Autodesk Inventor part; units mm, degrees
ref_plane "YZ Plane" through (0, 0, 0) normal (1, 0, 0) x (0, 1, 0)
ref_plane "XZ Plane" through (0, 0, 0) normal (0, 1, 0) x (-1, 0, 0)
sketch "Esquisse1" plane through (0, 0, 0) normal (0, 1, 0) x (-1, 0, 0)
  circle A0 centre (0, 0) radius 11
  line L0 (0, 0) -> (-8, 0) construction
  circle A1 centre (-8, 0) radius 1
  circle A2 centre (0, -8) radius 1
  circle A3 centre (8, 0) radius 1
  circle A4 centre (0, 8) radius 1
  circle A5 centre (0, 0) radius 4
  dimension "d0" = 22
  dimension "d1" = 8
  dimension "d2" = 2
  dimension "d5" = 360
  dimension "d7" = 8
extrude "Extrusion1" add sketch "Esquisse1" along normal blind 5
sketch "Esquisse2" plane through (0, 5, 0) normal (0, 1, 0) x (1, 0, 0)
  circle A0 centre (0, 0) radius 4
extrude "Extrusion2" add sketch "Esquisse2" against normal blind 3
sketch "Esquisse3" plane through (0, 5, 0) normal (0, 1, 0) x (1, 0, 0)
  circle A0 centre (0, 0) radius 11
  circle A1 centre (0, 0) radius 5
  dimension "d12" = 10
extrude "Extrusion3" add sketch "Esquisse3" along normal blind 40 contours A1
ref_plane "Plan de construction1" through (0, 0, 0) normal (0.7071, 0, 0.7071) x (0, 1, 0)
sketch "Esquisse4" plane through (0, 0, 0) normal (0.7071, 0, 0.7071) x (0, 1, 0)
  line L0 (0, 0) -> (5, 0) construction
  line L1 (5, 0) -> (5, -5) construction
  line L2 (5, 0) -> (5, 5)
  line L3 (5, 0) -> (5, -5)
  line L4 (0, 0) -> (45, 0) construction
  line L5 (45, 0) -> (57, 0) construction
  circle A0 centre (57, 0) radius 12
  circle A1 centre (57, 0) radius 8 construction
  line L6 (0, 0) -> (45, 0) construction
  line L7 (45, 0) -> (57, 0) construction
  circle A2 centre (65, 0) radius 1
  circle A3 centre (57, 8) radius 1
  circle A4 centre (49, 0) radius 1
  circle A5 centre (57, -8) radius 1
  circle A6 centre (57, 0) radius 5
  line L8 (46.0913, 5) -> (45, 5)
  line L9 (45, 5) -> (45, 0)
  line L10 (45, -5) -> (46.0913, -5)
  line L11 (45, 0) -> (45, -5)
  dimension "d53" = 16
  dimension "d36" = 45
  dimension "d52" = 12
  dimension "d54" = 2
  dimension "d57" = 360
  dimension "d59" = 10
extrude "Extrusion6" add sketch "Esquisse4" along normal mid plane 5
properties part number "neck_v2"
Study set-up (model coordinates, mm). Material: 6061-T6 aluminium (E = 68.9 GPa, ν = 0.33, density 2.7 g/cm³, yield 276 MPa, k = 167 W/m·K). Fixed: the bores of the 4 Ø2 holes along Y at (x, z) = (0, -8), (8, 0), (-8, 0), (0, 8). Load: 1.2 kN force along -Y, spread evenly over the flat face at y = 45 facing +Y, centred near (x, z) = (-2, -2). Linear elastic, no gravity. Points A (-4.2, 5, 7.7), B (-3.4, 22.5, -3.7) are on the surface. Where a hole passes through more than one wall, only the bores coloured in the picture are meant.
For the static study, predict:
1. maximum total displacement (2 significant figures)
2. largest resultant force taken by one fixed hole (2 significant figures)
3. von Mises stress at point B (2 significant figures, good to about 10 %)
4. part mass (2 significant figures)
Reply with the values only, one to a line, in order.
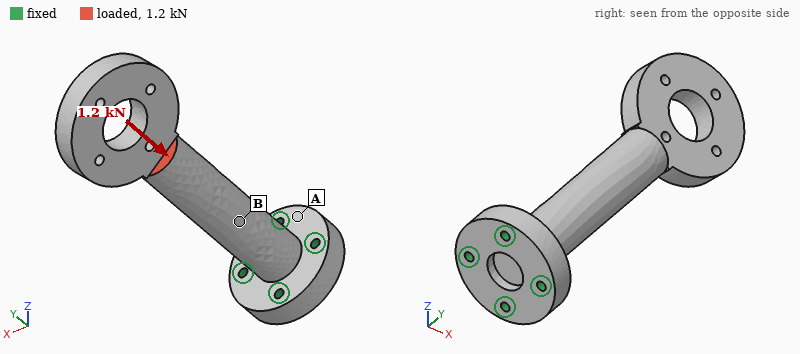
0.25 mm
520 N
58 MPa
18 g
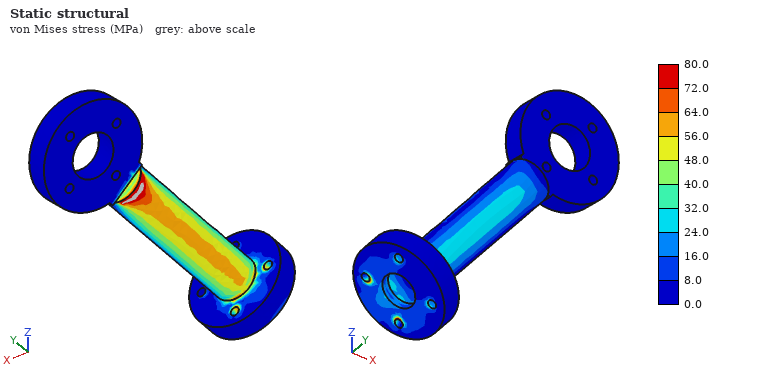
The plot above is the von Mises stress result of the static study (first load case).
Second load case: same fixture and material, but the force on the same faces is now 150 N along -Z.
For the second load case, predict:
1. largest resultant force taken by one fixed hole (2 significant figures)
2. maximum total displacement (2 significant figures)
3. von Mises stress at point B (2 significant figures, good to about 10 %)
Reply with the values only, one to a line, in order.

430 N
0.22 mm
26 MPa
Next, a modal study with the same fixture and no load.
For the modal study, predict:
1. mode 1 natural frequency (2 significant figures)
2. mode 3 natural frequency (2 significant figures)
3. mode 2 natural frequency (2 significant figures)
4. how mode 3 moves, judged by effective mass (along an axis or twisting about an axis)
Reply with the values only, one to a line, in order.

1500 Hz
6500 Hz
1500 Hz
twisting about Y
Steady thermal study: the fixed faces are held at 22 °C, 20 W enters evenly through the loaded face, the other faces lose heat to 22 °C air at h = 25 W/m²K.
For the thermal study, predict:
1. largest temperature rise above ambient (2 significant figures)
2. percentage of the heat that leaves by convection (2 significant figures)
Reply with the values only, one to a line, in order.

72 K
14 %
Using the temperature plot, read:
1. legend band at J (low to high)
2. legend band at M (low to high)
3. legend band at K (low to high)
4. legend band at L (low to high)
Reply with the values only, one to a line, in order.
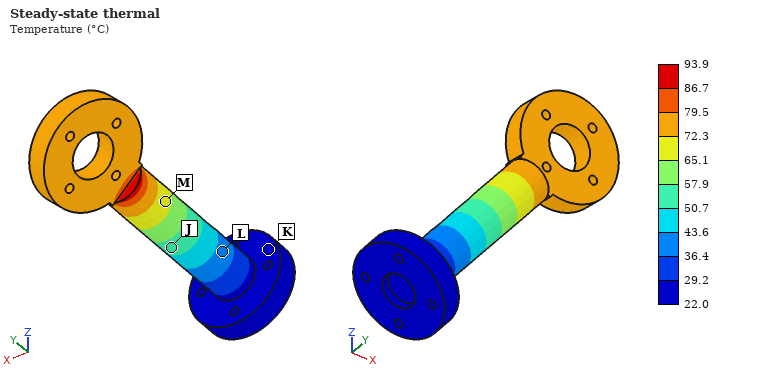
50.7 to 57.9 °C
65.1 to 72.3 °C
22.0 to 29.2 °C
36.4 to 43.6 °C
